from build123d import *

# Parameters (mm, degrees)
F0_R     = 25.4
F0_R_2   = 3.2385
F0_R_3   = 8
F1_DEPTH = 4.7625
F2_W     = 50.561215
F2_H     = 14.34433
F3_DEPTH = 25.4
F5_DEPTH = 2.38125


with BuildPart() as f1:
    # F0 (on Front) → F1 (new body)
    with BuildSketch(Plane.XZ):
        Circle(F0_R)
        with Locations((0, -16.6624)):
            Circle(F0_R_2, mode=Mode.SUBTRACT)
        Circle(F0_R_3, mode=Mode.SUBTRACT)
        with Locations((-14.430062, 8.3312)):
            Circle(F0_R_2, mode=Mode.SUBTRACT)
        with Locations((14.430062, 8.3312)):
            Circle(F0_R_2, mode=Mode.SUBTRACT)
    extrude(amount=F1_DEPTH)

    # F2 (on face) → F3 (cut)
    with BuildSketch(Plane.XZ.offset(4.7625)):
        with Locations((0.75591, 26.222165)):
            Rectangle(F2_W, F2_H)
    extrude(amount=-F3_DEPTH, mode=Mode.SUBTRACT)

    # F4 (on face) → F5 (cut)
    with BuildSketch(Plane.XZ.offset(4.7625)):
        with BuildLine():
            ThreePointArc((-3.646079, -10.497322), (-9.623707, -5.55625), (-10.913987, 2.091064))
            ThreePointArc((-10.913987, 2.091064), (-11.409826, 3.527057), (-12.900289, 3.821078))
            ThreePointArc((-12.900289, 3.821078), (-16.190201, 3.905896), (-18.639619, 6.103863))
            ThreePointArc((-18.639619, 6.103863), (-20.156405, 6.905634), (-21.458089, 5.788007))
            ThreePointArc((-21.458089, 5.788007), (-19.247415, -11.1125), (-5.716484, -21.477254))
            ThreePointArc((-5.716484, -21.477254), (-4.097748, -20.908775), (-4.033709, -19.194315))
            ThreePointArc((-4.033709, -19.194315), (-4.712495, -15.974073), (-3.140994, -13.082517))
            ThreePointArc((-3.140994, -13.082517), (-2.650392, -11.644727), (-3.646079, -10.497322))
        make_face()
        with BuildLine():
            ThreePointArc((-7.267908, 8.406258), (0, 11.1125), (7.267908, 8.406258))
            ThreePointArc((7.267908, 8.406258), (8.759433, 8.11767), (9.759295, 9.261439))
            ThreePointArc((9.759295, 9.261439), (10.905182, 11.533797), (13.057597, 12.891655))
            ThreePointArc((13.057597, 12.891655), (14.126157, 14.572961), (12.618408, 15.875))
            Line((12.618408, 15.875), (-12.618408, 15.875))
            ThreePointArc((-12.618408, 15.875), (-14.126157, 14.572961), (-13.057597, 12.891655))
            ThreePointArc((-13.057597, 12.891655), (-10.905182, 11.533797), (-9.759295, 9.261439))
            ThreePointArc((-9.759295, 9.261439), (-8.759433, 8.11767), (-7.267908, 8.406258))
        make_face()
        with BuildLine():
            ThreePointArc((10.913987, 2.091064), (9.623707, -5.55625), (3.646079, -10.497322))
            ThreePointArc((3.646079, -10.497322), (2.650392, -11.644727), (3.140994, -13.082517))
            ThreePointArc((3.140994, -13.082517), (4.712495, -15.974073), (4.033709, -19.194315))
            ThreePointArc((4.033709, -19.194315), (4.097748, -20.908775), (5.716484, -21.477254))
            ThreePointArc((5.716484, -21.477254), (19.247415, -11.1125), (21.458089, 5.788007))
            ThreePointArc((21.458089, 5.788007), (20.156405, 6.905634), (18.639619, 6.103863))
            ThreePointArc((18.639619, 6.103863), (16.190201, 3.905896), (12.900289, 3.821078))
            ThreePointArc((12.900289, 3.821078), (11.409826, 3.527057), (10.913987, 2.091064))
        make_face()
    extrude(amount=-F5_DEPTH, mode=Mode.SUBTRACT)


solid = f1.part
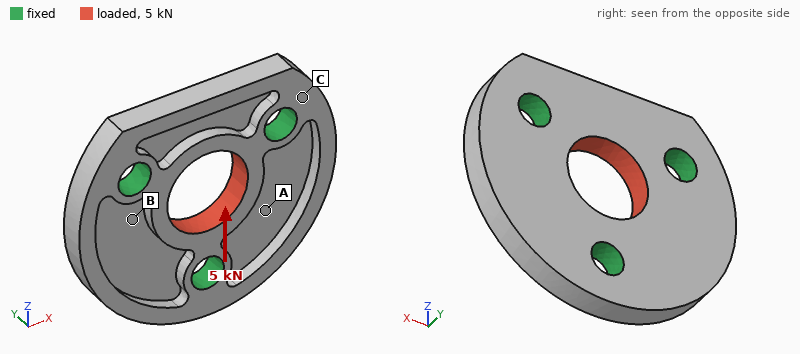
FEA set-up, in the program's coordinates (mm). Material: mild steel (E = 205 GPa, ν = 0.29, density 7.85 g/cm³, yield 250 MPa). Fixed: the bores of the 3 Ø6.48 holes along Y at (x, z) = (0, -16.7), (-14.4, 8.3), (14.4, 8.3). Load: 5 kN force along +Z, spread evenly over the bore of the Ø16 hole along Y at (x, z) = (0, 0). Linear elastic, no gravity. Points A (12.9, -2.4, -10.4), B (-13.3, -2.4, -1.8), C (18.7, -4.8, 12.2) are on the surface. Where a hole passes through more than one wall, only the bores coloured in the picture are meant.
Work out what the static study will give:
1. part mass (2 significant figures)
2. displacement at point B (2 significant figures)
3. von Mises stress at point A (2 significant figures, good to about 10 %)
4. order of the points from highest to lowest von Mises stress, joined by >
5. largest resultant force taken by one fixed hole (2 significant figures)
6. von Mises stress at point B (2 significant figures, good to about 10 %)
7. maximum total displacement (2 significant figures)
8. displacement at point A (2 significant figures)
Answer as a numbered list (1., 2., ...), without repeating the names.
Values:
1. 45 g
2. 1.3 µm
3. 14 MPa
4. B > A > C
5. 1.7 kN
6. 23 MPa
7. 5.6 µm
8. 1.5 µm
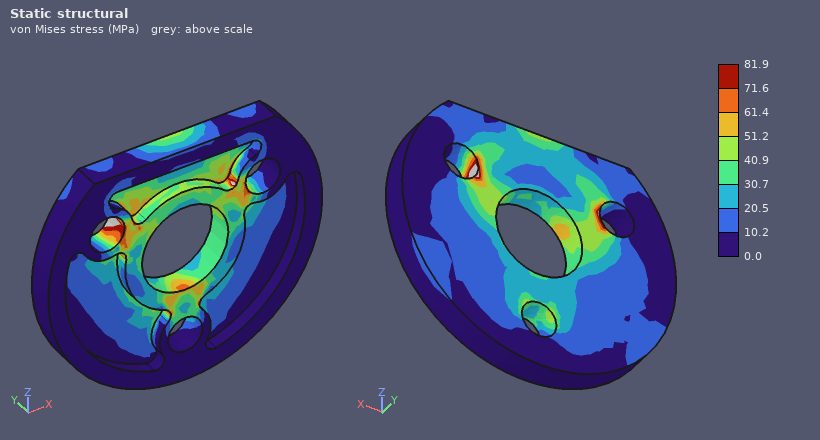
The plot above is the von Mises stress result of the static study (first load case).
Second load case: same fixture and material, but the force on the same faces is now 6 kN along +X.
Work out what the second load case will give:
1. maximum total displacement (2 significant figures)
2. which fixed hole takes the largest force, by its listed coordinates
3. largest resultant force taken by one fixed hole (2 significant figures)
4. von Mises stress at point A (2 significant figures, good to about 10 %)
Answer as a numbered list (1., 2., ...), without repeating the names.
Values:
1. 5.4 µm
2. (0, -16.7)
3. 2.2 kN
4. 25 MPa
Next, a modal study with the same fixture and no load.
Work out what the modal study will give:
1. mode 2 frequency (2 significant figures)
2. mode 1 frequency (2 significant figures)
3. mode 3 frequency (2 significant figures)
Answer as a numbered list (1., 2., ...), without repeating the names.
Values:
1. 11 kHz
2. 11 kHz
3. 21 kHz
